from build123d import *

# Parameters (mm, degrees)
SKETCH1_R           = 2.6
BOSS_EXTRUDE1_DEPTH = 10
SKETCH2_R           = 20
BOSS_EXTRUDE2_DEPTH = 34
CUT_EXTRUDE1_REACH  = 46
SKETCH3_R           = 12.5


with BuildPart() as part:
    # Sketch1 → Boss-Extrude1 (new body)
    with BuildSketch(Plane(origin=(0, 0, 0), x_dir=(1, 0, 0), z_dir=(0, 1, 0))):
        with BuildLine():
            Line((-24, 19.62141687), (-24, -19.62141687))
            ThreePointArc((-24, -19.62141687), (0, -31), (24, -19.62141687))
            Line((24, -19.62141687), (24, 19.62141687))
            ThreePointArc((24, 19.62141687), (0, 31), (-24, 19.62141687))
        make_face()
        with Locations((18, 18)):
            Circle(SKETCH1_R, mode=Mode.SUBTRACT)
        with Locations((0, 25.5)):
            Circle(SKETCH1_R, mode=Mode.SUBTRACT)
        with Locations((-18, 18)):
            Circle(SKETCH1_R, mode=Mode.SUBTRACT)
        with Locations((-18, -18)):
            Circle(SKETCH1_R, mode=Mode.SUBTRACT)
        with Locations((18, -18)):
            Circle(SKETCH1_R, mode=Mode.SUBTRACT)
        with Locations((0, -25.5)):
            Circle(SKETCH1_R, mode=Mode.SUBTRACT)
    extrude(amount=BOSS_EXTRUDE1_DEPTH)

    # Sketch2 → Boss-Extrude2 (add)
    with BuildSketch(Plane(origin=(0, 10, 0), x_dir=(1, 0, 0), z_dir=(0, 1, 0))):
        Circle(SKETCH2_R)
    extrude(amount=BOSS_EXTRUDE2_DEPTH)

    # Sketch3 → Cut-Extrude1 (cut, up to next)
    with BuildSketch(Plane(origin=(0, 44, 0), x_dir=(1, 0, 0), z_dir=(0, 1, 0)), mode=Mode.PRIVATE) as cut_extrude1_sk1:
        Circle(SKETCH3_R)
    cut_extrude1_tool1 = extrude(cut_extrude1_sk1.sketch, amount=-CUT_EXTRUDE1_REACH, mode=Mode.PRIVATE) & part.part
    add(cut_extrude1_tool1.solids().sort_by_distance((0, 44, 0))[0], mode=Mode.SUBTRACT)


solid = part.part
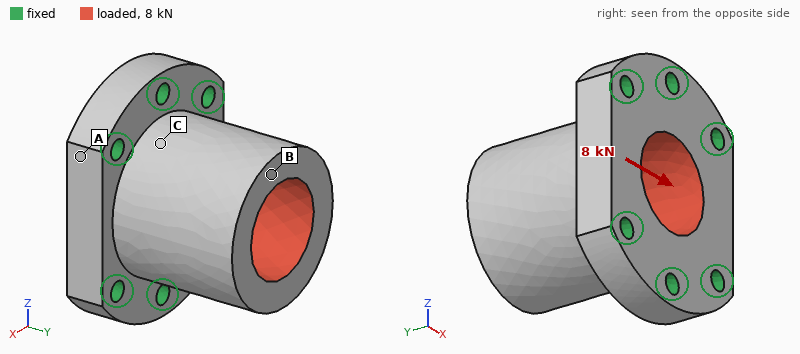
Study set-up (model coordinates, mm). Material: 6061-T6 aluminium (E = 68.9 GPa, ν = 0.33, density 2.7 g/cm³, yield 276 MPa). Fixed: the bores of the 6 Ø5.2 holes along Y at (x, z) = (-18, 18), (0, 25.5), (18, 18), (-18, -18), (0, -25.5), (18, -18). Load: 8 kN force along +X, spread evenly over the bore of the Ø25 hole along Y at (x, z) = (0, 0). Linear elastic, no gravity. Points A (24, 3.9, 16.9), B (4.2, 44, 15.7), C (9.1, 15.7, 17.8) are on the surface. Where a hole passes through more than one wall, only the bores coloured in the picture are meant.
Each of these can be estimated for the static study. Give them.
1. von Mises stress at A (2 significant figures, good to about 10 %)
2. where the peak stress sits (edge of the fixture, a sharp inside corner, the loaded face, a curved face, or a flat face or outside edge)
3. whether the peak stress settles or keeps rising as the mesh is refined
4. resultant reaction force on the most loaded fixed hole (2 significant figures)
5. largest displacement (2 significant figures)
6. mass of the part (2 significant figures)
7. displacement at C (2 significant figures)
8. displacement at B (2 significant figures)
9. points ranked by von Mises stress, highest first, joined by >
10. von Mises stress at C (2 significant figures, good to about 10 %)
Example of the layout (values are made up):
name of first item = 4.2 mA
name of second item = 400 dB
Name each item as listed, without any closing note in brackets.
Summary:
von Mises stress at A = 11 MPa
where the peak stress sits = edge of the fixture
whether the peak stress settles or keeps rising as the mesh is refined = keeps rising
resultant reaction force on the most loaded fixed hole = 2.6 kN
largest displacement = 30 µm
mass of the part = 120 g
displacement at C = 8.3 µm
displacement at B = 27 µm
points ranked by von Mises stress, highest first, joined by > = C > A > B
von Mises stress at C = 17 MPa
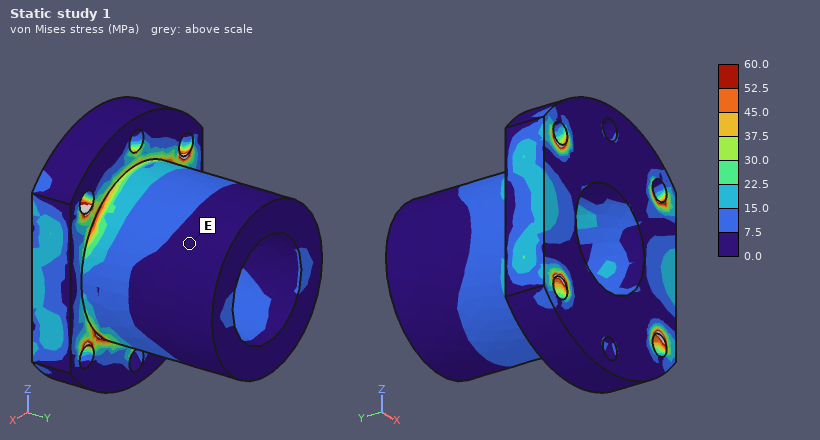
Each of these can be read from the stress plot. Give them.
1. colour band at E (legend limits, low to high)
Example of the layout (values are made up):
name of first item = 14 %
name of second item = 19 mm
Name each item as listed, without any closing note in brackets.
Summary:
colour band at E = 0.0 to 7.5 MPa
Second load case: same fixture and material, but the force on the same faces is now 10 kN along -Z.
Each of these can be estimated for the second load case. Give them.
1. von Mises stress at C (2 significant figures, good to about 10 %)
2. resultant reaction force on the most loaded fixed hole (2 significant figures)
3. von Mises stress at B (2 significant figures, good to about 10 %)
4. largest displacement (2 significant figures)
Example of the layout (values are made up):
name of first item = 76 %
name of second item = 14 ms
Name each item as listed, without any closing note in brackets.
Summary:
von Mises stress at C = 17 MPa
resultant reaction force on the most loaded fixed hole = 2.6 kN
von Mises stress at B = 9.1 MPa
largest displacement = 27 µm
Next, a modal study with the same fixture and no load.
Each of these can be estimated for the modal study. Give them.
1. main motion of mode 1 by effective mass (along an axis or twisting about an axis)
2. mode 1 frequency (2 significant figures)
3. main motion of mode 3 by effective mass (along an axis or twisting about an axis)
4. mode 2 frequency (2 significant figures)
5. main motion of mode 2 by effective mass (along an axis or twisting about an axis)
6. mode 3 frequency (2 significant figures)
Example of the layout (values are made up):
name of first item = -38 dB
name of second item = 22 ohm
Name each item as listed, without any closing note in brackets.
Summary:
main motion of mode 1 by effective mass = along X
mode 1 frequency = 10 kHz
main motion of mode 3 by effective mass = along Y
mode 2 frequency = 12 kHz
main motion of mode 2 by effective mass = along Z
mode 3 frequency = 18 kHz
